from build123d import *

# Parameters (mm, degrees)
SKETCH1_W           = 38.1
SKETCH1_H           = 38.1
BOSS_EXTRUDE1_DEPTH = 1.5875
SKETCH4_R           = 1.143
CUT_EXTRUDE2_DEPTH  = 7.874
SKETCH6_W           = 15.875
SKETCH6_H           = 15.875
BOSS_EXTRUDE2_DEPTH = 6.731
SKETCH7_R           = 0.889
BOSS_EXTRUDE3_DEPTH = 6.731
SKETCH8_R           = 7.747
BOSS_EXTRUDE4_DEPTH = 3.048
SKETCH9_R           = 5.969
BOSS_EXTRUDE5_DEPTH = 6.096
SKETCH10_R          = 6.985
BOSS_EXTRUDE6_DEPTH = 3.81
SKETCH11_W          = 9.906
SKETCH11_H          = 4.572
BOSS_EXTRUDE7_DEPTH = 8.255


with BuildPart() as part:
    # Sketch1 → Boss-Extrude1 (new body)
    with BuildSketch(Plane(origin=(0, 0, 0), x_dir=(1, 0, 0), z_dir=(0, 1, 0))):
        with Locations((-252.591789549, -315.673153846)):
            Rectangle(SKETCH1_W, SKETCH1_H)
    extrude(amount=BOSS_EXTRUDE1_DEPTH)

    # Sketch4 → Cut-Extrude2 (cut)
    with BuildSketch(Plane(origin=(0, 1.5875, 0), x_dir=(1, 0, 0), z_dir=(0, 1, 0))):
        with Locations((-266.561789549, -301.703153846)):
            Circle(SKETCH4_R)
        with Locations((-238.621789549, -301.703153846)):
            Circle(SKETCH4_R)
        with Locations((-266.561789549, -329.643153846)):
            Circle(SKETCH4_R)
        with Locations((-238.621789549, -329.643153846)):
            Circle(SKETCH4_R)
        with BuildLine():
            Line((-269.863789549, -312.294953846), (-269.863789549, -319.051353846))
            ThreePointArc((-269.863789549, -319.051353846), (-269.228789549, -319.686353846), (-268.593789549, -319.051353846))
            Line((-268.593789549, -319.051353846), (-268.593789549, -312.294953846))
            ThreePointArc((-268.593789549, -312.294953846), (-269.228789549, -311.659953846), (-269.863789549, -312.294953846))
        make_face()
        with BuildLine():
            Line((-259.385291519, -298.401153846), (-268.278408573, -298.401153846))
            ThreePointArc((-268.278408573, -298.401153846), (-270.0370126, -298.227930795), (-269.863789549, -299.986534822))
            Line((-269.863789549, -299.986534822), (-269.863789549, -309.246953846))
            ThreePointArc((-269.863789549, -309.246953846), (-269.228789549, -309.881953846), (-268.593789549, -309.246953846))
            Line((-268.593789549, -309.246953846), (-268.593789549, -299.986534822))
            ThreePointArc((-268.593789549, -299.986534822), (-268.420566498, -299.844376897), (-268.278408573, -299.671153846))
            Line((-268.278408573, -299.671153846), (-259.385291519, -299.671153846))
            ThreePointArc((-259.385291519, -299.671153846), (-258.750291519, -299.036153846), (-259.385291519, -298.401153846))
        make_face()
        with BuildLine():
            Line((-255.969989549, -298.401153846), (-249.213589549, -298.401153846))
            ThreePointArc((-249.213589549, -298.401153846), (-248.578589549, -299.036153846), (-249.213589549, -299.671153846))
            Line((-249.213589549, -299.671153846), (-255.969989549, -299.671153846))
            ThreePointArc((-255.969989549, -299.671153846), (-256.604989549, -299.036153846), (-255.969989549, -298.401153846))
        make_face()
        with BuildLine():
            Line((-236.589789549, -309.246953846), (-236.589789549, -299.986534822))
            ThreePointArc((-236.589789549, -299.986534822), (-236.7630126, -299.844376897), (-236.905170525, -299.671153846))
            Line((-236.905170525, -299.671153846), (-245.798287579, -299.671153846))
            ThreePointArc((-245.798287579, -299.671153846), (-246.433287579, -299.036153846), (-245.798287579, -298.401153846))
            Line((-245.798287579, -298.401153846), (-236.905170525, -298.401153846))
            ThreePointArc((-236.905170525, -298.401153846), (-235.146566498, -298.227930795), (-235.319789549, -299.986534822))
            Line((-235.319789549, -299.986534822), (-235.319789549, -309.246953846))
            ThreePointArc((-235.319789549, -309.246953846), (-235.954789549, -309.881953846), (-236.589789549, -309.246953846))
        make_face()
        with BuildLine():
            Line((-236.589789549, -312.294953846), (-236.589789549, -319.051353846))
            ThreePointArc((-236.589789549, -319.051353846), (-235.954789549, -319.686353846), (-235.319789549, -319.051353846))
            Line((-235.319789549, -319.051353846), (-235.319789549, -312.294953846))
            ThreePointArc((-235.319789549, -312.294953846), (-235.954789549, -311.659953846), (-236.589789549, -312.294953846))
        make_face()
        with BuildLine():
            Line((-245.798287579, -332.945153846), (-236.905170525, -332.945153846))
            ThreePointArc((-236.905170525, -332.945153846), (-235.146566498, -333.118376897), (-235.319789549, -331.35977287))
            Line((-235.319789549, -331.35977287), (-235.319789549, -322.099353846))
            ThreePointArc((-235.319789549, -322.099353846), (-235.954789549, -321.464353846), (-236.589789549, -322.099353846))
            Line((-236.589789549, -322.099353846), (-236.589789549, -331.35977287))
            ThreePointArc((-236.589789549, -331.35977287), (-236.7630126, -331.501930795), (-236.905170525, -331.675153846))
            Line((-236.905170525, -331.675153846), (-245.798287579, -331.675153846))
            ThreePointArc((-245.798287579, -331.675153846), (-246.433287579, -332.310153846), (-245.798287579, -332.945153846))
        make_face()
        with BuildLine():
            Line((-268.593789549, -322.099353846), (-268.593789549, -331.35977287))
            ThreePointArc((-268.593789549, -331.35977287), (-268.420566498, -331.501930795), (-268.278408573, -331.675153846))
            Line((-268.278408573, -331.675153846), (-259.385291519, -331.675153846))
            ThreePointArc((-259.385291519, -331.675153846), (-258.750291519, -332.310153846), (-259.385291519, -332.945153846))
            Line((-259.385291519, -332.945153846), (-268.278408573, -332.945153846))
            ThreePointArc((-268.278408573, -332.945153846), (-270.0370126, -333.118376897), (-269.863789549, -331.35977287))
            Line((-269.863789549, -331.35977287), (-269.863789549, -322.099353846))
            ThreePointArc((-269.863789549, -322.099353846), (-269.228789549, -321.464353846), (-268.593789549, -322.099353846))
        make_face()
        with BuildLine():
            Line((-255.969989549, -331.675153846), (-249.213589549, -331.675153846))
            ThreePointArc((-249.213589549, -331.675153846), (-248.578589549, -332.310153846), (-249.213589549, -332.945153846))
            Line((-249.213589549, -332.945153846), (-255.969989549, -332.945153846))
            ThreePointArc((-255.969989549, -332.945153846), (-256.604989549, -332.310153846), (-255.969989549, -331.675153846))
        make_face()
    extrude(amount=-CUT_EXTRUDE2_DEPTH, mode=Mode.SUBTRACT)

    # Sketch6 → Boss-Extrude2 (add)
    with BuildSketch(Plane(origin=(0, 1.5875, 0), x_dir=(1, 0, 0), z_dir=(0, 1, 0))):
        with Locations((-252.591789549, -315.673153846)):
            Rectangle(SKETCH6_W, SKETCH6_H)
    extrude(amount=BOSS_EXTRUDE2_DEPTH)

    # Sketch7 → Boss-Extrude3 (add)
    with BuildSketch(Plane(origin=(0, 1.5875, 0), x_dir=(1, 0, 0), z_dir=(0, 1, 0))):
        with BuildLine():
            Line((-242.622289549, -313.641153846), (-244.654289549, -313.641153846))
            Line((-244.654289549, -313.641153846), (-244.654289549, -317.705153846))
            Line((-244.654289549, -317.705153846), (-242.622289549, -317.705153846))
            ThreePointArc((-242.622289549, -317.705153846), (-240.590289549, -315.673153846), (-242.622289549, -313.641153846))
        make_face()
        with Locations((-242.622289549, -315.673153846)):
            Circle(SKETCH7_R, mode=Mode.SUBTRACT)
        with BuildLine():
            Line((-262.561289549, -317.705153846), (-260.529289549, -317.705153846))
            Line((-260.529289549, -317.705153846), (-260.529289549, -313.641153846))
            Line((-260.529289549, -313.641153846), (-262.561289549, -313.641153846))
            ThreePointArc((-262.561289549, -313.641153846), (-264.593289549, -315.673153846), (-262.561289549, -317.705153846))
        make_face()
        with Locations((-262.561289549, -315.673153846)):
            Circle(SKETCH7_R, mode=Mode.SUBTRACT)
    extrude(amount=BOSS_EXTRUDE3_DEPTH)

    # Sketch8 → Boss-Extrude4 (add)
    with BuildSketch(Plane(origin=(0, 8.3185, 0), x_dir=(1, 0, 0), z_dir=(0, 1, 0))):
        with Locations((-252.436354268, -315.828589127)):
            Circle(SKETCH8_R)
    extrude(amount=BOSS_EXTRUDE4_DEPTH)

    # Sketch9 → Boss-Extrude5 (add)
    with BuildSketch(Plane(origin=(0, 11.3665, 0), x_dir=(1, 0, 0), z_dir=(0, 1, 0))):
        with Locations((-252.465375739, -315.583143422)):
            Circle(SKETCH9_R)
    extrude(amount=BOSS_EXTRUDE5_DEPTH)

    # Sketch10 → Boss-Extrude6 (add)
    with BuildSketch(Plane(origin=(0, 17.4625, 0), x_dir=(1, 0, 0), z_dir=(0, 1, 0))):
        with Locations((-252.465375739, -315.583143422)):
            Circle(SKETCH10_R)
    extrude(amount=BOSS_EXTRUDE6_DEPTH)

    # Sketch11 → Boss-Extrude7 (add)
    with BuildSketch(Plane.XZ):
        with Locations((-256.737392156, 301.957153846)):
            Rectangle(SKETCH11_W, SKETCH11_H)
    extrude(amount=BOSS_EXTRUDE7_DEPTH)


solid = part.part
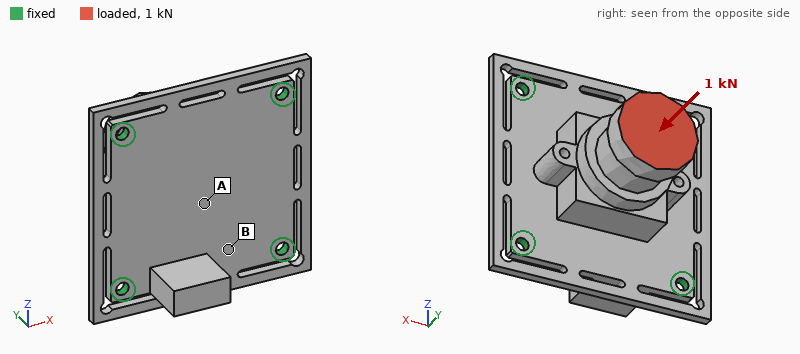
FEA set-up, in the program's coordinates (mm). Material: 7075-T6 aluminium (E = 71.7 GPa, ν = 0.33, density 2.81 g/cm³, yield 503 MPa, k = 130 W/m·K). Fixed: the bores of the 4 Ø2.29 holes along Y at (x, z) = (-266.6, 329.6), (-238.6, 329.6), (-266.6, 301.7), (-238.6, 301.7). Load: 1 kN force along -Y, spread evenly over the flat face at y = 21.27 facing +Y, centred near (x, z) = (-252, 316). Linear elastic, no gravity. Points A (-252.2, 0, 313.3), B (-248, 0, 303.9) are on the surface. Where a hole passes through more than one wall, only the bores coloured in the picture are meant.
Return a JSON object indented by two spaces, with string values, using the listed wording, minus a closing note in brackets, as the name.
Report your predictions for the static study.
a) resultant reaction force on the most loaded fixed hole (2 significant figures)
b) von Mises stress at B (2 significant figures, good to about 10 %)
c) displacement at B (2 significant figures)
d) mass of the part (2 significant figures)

{
  "resultant reaction force on the most loaded fixed hole": "270 N",
  "von Mises stress at B": "77 MPa",
  "displacement at B": "63 µm",
  "mass of the part": "17 g"
}
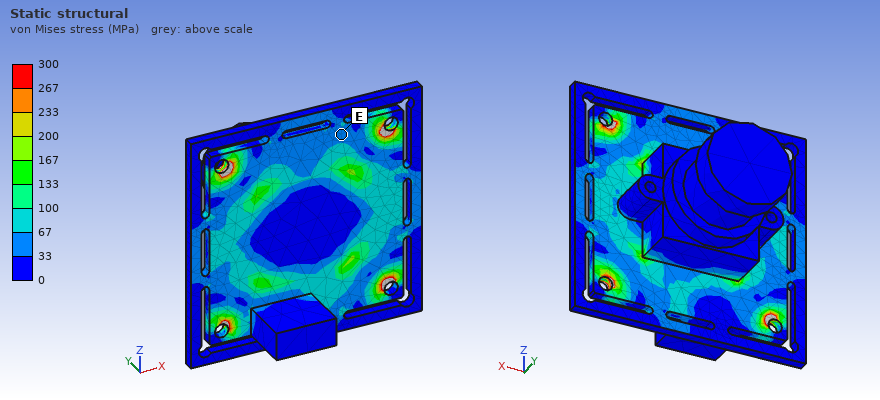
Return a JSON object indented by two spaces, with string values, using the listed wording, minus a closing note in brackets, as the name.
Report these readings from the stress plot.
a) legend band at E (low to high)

{
  "legend band at E": "33 to 67 MPa"
}
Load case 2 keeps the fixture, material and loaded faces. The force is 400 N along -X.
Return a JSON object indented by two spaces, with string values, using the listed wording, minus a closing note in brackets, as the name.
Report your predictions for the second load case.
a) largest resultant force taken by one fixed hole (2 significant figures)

{
  "largest resultant force taken by one fixed hole": "220 N"
}
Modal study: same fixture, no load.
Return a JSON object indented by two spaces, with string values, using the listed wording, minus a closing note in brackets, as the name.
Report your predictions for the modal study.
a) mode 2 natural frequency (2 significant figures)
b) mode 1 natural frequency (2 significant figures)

{
  "mode 2 natural frequency": "4800 Hz",
  "mode 1 natural frequency": "4700 Hz"
}
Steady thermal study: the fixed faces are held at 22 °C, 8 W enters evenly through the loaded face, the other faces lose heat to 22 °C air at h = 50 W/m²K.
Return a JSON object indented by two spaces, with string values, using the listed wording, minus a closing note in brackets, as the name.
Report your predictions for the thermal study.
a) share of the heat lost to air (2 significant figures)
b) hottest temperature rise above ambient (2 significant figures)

{
  "share of the heat lost to air": "19 %",
  "hottest temperature rise above ambient": "16 K"
}
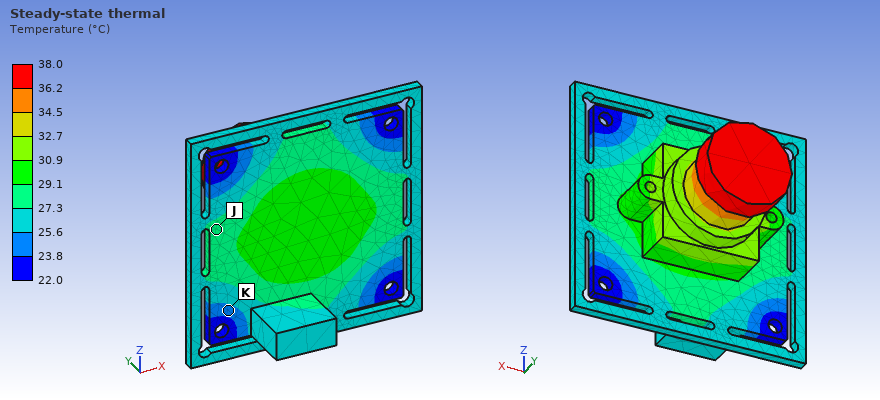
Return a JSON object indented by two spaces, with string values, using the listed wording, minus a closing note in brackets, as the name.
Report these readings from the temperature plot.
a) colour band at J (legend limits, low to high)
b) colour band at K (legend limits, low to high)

{
  "colour band at J": "27.3 to 29.1 °C",
  "colour band at K": "23.8 to 25.6 °C"
}
